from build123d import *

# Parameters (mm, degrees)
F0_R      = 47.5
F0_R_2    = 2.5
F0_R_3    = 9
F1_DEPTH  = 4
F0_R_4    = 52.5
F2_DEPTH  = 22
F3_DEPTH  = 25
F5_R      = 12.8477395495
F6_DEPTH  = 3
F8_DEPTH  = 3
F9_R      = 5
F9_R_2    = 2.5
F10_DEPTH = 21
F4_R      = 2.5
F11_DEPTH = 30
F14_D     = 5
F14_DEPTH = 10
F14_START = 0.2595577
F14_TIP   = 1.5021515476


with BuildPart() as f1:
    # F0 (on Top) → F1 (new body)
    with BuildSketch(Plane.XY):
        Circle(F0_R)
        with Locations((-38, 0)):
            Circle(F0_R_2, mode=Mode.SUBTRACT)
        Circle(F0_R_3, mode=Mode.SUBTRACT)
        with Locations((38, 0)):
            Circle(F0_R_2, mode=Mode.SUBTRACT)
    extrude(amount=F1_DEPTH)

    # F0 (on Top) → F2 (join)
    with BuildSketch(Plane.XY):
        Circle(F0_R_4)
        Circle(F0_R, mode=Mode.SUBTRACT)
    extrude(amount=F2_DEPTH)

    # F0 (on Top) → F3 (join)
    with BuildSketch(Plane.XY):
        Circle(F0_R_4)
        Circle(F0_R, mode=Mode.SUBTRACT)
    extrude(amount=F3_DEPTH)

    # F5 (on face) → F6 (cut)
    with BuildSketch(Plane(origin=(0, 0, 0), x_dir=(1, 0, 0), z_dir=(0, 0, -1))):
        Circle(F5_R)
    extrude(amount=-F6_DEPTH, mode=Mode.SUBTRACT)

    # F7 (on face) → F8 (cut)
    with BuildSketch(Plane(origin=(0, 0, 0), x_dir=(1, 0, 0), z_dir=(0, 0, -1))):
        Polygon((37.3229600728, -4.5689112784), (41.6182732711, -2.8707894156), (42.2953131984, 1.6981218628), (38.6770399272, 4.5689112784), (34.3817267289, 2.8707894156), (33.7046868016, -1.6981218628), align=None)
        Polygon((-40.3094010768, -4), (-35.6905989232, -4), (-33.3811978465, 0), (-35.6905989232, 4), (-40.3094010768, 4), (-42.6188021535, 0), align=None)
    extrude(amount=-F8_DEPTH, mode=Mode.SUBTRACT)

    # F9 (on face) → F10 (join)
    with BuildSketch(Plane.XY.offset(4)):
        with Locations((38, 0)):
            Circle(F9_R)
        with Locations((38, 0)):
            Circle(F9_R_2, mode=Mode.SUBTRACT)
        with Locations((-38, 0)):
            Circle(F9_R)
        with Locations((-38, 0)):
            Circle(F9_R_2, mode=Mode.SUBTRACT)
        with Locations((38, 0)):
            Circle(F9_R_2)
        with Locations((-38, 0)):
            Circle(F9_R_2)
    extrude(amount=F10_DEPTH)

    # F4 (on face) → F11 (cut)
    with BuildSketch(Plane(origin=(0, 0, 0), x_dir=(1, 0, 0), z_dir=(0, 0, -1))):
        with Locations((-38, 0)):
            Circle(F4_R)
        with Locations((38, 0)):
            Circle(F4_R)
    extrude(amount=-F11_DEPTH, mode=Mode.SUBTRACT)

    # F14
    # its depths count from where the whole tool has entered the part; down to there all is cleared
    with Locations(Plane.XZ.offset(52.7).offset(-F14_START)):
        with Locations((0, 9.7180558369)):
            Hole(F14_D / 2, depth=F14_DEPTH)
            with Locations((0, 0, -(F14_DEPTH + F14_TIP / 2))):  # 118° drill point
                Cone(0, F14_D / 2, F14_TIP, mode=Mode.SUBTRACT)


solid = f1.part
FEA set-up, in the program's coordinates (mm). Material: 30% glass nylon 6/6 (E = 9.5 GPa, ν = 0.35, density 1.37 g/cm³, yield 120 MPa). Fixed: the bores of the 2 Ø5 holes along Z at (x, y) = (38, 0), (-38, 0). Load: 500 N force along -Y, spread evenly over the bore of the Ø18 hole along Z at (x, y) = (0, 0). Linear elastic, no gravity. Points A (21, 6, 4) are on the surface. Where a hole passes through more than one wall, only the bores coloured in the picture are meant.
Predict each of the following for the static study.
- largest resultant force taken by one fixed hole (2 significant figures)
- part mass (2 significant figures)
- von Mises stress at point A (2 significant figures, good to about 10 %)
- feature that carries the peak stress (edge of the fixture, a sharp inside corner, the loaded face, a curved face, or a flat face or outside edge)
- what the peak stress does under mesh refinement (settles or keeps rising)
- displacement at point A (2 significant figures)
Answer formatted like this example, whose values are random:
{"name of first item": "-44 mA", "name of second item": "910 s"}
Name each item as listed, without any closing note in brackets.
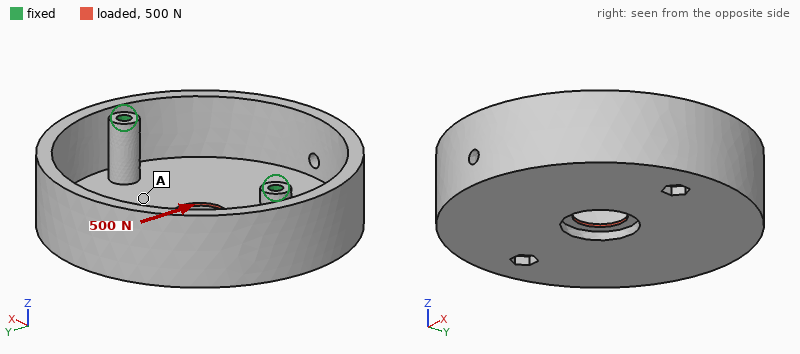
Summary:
{"largest resultant force taken by one fixed hole": "250 N", "part mass": "93 g", "von Mises stress at point A": "1.7 MPa", "feature that carries the peak stress": "a sharp inside corner", "what the peak stress does under mesh refinement": "keeps rising", "displacement at point A": "9.3 µm"}
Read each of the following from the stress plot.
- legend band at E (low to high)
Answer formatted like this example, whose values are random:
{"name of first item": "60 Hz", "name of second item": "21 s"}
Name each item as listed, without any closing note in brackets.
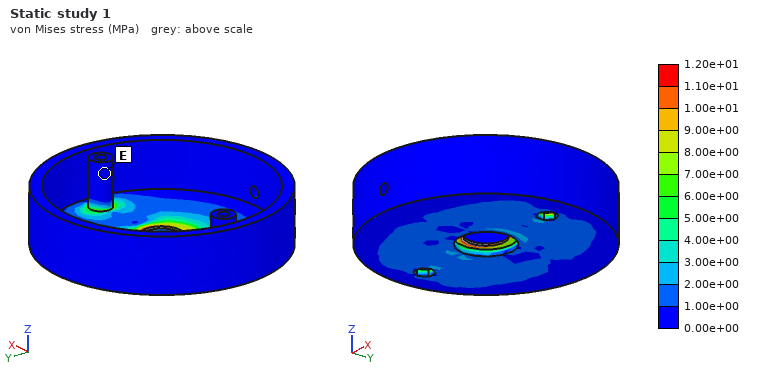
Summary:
{"legend band at E": "0.00e+00 to 1.00e+00 MPa"}
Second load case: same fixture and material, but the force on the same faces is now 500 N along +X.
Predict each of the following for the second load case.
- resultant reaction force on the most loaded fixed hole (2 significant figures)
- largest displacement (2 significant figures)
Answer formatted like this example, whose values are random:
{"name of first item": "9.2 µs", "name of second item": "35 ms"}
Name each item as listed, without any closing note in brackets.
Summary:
{"resultant reaction force on the most loaded fixed hole": "250 N", "largest displacement": "19 µm"}
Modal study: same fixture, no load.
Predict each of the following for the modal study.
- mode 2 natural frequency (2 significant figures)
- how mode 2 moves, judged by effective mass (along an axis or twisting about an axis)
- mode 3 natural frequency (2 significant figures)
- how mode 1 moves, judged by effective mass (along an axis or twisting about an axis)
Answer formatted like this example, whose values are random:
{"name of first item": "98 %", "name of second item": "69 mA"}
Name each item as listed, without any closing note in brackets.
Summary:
{"mode 2 natural frequency": "1100 Hz", "how mode 2 moves, judged by effective mass": "along Z", "mode 3 natural frequency": "1400 Hz", "how mode 1 moves, judged by effective mass": "twisting about X"}
